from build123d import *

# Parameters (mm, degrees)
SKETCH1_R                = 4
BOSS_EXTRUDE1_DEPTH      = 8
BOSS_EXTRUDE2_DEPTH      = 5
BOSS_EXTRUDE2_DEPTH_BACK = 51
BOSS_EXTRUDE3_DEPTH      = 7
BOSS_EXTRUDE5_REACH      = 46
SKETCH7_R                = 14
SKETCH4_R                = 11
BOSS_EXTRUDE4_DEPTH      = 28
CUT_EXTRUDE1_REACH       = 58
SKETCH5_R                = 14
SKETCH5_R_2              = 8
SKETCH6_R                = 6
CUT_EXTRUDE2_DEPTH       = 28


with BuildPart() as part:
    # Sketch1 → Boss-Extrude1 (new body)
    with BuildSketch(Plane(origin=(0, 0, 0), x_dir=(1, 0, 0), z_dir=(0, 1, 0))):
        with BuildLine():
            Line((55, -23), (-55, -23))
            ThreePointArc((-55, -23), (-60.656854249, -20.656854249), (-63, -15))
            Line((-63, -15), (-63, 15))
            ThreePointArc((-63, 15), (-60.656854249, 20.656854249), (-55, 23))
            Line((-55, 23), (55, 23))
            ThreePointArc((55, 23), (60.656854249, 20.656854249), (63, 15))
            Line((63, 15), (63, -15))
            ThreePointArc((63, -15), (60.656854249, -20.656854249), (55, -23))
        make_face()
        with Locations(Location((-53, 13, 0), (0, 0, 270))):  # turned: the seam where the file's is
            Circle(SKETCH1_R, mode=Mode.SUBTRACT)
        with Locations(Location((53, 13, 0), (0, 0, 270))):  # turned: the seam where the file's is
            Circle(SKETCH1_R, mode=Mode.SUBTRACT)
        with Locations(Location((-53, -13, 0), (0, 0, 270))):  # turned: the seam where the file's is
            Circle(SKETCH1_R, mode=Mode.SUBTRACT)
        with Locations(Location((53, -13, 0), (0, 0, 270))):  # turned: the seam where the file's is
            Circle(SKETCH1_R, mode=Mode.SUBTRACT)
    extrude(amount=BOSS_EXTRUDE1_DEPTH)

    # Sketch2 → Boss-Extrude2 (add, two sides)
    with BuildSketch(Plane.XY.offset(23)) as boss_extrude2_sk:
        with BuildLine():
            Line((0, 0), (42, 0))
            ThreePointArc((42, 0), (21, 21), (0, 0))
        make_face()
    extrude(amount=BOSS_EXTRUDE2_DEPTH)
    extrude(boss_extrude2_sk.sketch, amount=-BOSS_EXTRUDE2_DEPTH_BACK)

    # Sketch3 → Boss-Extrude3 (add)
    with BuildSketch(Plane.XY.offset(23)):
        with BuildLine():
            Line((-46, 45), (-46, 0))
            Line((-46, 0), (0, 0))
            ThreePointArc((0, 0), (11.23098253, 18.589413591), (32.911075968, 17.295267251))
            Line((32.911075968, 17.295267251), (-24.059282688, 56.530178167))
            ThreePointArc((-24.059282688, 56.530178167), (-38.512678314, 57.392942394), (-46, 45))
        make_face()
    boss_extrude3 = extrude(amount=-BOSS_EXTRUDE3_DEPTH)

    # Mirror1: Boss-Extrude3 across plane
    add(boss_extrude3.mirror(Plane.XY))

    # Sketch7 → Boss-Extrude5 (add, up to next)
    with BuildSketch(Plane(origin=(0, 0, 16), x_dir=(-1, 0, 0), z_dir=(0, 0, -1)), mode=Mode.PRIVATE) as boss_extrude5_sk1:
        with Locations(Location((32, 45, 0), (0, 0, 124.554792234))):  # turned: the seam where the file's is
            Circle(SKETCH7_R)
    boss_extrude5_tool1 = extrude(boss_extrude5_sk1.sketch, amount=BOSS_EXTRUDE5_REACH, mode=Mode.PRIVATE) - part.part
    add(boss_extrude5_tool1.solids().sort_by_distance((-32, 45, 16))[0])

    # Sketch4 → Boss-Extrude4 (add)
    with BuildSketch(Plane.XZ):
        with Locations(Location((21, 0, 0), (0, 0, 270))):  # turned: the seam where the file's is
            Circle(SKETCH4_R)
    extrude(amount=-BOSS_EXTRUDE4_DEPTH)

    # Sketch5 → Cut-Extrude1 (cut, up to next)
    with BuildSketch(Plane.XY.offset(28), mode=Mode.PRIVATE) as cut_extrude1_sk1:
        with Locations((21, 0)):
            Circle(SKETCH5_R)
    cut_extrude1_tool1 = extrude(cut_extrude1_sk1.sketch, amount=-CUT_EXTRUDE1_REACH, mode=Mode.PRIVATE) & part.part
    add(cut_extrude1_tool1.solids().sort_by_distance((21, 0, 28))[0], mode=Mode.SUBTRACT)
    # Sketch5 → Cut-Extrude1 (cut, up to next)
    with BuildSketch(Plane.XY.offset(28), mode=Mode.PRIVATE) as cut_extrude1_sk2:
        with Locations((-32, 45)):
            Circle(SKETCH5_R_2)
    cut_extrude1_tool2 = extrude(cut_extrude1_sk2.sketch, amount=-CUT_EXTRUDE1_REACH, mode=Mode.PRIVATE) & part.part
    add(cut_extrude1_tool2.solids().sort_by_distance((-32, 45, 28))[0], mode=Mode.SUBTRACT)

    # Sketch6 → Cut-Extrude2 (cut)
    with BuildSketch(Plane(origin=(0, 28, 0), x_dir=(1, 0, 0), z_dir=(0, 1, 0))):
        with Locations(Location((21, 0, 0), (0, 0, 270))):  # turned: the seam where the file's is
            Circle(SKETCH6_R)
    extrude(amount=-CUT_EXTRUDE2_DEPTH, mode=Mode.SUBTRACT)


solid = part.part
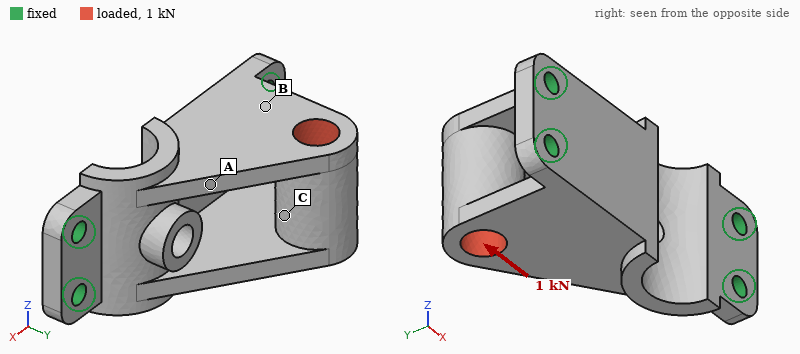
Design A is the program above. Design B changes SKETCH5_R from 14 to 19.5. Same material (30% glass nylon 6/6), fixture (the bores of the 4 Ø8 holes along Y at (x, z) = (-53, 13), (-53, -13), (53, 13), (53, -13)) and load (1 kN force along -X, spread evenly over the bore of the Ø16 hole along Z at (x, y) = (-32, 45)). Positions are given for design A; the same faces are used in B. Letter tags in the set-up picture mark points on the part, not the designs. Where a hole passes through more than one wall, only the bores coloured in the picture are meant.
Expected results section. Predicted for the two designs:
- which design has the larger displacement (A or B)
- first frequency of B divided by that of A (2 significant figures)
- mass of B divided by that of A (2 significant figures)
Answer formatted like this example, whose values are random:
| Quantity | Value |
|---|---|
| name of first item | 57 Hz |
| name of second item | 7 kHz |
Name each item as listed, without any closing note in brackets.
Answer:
| Quantity | Value |
|---|---|
| which design has the larger displacement | B |
| first frequency of B divided by that of A | 0.90 |
| mass of B divided by that of A | 0.84 |
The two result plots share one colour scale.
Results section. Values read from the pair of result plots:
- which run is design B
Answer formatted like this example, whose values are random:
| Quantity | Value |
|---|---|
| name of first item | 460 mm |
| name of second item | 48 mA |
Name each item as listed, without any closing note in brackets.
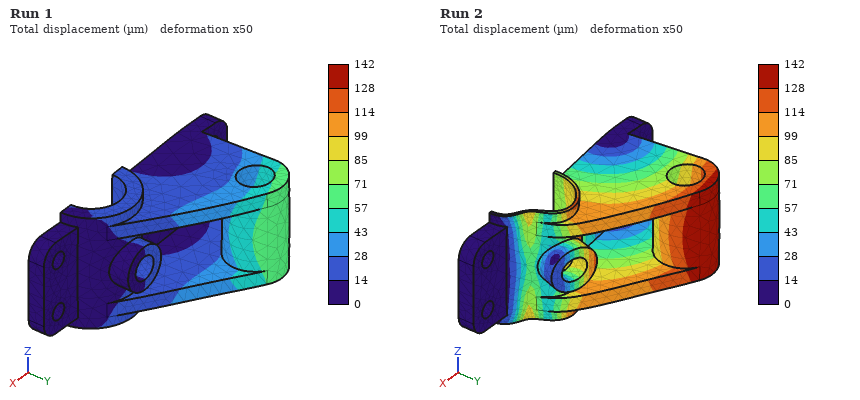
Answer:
| Quantity | Value |
|---|---|
| which run is design B | Run 2 |
